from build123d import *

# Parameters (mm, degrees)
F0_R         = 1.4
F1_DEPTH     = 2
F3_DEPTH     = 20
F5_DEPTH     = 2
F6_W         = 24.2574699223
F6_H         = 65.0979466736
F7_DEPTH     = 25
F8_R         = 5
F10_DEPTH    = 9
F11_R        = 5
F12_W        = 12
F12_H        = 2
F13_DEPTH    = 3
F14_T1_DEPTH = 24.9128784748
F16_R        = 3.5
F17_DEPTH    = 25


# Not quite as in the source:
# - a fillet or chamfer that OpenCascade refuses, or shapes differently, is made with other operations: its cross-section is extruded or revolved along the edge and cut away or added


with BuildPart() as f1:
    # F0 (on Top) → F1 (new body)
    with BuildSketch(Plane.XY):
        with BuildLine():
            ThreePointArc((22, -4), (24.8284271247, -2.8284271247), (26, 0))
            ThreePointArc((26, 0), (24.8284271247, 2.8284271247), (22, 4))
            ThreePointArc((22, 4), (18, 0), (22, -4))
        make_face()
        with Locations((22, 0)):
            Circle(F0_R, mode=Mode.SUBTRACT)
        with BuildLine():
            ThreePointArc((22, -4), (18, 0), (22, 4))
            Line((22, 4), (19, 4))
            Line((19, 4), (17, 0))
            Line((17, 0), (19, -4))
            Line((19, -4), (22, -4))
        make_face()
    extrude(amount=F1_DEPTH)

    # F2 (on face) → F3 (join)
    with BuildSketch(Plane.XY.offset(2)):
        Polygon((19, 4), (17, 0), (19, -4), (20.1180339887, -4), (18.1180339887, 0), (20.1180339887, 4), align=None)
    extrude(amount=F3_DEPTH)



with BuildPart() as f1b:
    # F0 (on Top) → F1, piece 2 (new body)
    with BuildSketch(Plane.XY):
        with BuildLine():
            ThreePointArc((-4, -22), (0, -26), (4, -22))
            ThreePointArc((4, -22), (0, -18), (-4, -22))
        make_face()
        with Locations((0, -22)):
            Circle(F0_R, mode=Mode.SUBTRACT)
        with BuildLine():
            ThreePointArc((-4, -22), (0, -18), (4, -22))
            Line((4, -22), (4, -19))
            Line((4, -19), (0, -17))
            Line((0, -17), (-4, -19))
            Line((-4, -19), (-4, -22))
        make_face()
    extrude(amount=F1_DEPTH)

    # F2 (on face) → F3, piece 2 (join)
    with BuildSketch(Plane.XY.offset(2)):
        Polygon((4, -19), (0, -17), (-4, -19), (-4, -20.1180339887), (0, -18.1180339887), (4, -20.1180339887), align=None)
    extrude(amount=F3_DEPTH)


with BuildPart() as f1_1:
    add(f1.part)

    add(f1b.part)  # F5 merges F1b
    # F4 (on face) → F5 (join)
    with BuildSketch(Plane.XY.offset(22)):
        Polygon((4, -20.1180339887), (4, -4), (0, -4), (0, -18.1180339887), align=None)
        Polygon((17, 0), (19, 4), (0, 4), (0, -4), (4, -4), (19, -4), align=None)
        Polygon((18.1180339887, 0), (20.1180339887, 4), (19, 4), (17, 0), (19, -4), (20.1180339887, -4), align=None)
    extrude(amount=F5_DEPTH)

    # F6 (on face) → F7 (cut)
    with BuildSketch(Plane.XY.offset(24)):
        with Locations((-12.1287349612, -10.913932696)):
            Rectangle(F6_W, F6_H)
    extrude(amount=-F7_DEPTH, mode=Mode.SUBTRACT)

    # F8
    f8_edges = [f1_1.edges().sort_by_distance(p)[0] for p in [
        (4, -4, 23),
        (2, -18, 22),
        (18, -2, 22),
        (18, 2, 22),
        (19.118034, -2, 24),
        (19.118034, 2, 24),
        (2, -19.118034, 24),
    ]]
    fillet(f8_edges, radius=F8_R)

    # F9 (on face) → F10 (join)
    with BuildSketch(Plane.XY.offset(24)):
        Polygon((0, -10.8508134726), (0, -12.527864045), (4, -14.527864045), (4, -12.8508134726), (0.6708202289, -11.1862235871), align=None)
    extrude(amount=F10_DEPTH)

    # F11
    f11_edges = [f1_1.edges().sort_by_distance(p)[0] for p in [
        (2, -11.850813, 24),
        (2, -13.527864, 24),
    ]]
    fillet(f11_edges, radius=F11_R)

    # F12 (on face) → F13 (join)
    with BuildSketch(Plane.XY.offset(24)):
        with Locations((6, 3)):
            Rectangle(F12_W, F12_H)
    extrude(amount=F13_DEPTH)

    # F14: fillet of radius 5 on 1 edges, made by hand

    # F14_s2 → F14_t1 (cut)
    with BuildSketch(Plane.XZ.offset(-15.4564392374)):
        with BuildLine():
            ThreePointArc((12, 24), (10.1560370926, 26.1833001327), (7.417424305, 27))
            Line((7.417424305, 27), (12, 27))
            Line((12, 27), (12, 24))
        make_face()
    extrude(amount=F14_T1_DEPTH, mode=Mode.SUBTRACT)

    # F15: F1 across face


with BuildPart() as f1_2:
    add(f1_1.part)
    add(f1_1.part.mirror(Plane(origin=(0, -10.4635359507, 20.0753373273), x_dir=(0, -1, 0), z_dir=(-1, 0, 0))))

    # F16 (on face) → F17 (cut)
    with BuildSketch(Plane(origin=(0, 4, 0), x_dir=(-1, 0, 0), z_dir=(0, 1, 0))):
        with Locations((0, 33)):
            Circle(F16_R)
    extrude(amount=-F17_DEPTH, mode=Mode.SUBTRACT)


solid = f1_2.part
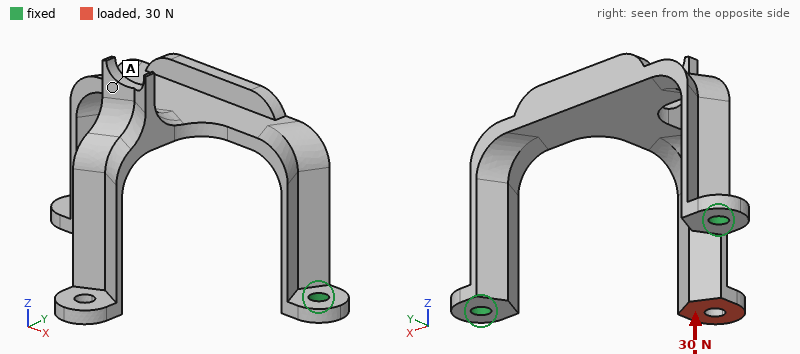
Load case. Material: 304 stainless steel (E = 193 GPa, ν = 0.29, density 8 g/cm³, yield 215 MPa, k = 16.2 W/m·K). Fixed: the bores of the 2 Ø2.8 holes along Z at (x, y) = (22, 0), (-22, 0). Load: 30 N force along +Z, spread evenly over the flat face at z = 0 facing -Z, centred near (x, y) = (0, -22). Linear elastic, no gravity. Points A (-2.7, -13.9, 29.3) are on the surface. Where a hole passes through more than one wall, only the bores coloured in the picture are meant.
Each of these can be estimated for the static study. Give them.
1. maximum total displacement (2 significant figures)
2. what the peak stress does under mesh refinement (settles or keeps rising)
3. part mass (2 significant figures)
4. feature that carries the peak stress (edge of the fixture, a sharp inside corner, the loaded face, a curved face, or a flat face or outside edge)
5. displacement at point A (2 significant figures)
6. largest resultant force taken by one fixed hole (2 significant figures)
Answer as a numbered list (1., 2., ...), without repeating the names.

1. 0.25 mm
2. keeps rising
3. 16 g
4. edge of the fixture
5. 0.10 mm
6. 16 N
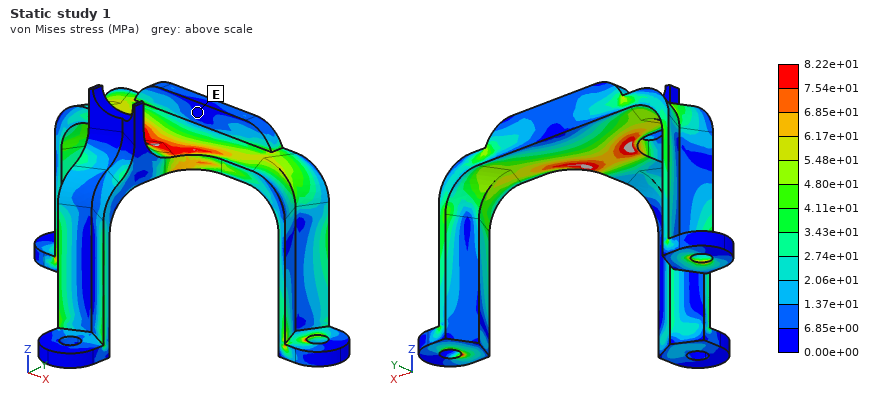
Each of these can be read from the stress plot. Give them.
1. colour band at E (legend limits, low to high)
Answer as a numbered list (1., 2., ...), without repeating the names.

1. 0.00e+00 to 6.85e+00 MPa
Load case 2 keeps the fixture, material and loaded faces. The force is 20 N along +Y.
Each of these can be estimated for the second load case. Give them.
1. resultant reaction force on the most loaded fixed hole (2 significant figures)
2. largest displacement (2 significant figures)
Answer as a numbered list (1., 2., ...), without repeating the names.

1. 10 N
2. 0.26 mm
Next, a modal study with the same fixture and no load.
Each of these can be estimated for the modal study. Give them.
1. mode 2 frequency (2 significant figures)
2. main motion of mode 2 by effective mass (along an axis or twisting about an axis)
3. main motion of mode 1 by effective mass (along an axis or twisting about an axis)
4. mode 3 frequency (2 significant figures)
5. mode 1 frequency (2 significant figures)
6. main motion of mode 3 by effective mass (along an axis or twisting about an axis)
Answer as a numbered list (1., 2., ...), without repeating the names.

1. 1400 Hz
2. along X
3. along Z
4. 2000 Hz
5. 1100 Hz
6. along Y
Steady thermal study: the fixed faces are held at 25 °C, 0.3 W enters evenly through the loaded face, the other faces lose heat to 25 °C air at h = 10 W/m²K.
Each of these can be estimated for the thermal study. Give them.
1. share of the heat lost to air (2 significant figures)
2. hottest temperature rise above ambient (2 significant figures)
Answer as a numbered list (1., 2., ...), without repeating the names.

1. 82 %
2. 43 K
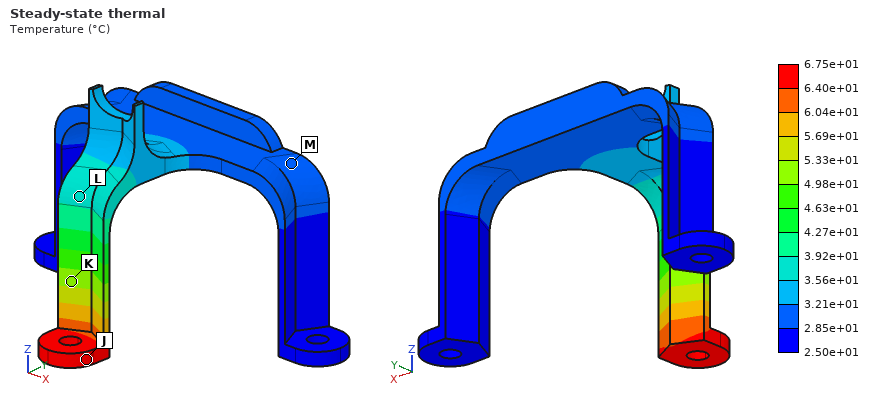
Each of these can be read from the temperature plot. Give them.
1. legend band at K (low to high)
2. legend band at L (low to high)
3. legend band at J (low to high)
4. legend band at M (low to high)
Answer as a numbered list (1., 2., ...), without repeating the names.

1. 4.98e+01 to 5.33e+01 °C
2. 3.56e+01 to 3.92e+01 °C
3. 6.40e+01 to 6.75e+01 °C
4. 2.85e+01 to 3.21e+01 °C
